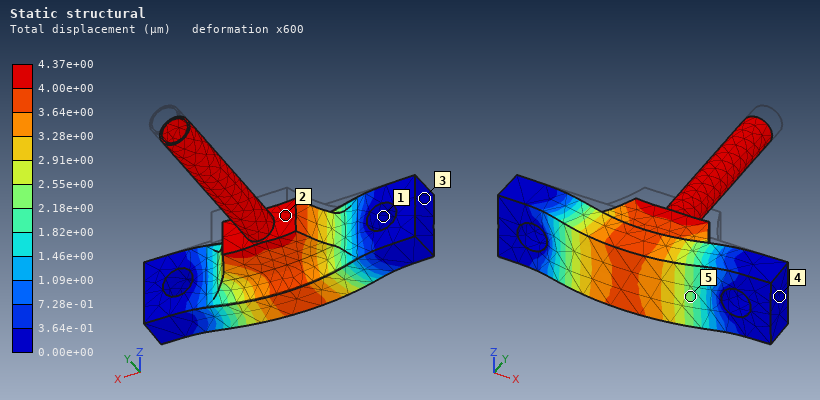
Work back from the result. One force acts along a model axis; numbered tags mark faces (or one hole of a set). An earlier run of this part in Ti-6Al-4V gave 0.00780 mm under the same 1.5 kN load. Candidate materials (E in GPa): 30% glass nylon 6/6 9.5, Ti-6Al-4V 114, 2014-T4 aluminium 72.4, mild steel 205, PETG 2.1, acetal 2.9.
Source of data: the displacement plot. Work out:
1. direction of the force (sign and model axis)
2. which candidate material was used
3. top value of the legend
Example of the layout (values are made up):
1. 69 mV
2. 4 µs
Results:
1. -Y
2. mild steel
3. 4.37e+00 µm
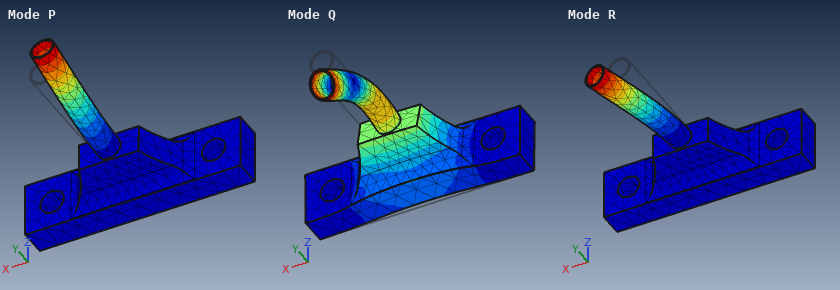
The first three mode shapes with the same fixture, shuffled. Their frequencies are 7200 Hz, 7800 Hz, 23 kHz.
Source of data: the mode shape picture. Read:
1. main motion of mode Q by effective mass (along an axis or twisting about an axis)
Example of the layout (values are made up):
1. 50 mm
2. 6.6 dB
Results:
1. along Z
